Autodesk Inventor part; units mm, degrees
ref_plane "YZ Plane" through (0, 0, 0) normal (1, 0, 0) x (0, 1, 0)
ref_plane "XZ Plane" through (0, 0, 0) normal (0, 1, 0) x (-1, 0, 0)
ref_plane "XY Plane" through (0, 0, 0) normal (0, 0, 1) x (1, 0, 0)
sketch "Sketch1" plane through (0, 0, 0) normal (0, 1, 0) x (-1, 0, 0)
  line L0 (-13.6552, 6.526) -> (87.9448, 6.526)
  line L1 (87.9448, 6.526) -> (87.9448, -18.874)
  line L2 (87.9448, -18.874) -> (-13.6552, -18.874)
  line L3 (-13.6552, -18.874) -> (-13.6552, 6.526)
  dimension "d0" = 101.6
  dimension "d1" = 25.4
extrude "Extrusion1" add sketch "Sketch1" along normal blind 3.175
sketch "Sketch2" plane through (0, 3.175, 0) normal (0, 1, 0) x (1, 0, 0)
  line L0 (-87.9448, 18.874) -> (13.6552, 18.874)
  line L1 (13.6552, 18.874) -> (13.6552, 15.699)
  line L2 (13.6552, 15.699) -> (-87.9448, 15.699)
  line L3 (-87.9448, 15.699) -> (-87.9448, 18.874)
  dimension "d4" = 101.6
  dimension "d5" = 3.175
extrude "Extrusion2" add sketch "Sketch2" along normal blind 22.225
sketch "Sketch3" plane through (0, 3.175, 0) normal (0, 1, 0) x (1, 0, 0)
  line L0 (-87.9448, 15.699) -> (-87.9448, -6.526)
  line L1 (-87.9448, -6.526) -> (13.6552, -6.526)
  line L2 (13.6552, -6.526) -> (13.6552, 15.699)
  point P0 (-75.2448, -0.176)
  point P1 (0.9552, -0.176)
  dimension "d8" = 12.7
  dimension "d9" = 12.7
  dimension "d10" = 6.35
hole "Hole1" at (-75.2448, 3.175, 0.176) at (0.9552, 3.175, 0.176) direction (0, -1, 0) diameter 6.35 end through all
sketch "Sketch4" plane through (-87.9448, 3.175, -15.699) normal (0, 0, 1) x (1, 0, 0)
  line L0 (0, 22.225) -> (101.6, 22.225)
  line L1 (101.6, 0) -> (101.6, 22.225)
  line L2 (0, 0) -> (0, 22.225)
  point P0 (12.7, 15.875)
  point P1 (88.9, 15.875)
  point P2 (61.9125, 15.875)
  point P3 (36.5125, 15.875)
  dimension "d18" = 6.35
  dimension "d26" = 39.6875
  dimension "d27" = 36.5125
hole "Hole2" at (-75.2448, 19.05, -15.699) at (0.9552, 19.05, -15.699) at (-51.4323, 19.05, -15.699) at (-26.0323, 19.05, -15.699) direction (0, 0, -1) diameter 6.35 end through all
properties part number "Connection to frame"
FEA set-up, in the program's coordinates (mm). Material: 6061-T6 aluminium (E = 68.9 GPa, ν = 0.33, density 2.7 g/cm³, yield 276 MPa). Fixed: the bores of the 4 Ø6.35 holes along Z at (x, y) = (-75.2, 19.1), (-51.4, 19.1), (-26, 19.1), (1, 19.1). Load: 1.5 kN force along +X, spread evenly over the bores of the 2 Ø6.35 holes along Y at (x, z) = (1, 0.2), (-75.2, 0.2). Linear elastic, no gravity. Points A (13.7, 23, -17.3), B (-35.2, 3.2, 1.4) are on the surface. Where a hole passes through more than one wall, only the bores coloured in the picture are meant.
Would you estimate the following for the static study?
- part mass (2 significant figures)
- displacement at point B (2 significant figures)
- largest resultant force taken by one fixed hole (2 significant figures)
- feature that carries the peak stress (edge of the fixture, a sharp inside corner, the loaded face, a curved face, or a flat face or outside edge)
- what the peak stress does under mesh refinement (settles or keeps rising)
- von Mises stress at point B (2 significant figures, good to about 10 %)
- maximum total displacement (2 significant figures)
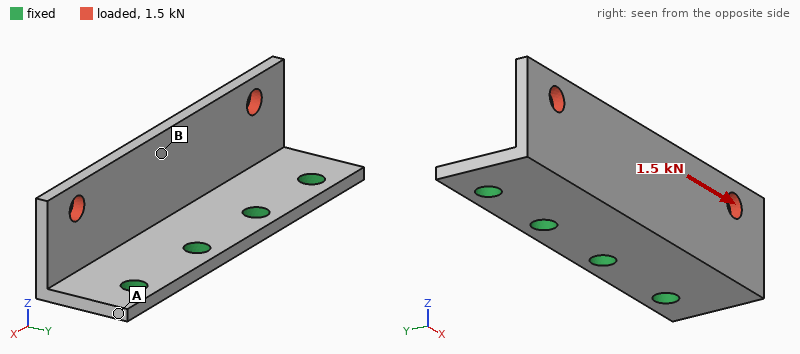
40 g
0.039 mm
530 N
edge of the fixture
keeps rising
21 MPa
0.15 mm
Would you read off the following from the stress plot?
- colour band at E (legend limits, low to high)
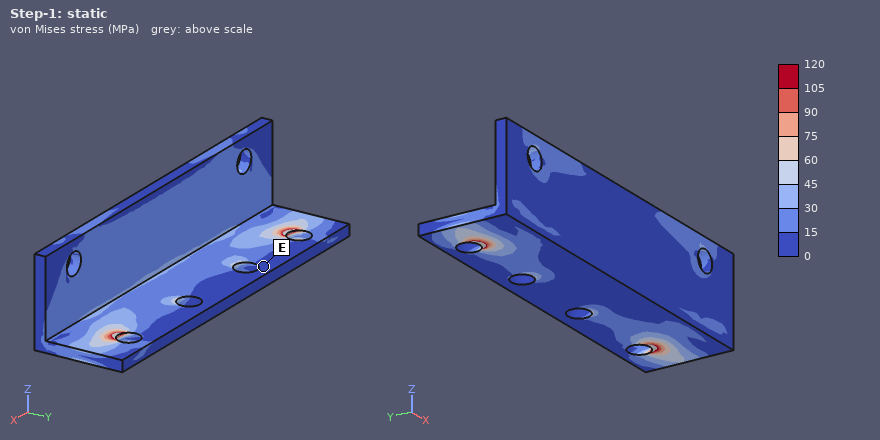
0 to 15 MPa
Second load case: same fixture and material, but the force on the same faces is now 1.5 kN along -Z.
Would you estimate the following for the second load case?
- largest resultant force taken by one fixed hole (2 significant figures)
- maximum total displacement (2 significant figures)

460 N
0.29 mm
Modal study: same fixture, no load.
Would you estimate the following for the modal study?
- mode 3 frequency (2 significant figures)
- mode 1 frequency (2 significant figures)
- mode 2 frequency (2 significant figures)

5900 Hz
2200 Hz
2900 Hz
